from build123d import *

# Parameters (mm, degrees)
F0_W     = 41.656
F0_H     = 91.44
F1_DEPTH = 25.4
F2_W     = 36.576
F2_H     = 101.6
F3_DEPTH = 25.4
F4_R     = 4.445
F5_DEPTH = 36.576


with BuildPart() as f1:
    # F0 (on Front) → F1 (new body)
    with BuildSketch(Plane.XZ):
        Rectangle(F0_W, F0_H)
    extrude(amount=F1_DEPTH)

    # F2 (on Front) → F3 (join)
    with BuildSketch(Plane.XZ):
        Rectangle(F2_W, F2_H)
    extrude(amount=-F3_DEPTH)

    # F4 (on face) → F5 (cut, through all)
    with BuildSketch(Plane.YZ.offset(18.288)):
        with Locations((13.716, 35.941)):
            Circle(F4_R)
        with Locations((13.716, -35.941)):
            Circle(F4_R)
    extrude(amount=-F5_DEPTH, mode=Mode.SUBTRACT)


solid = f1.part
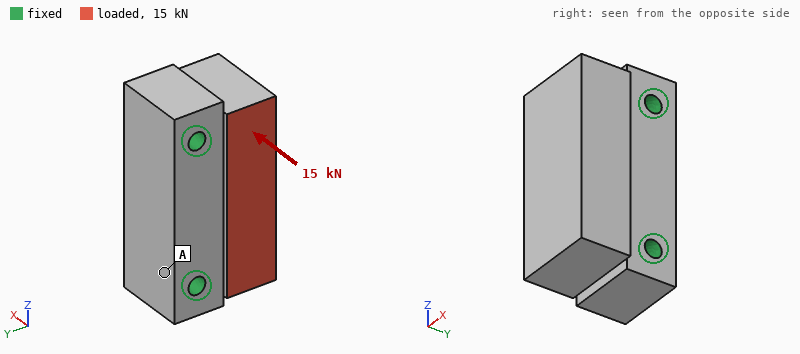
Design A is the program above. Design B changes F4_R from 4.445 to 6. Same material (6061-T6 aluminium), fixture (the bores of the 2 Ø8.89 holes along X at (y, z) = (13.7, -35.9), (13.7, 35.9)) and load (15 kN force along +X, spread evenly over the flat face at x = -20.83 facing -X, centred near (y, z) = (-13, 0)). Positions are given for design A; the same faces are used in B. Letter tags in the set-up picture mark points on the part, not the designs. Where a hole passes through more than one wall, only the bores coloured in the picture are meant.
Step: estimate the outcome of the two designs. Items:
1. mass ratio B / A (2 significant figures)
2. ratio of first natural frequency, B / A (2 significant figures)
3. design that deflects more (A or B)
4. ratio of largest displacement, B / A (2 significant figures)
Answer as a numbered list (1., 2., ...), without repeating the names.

1. 0.98
2. 1.1
3. A
4. 0.85
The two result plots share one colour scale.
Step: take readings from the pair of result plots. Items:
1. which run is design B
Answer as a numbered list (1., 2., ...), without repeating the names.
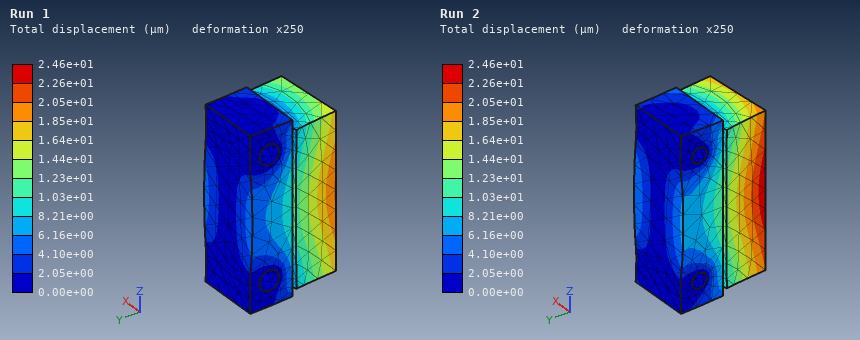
1. Run 1
